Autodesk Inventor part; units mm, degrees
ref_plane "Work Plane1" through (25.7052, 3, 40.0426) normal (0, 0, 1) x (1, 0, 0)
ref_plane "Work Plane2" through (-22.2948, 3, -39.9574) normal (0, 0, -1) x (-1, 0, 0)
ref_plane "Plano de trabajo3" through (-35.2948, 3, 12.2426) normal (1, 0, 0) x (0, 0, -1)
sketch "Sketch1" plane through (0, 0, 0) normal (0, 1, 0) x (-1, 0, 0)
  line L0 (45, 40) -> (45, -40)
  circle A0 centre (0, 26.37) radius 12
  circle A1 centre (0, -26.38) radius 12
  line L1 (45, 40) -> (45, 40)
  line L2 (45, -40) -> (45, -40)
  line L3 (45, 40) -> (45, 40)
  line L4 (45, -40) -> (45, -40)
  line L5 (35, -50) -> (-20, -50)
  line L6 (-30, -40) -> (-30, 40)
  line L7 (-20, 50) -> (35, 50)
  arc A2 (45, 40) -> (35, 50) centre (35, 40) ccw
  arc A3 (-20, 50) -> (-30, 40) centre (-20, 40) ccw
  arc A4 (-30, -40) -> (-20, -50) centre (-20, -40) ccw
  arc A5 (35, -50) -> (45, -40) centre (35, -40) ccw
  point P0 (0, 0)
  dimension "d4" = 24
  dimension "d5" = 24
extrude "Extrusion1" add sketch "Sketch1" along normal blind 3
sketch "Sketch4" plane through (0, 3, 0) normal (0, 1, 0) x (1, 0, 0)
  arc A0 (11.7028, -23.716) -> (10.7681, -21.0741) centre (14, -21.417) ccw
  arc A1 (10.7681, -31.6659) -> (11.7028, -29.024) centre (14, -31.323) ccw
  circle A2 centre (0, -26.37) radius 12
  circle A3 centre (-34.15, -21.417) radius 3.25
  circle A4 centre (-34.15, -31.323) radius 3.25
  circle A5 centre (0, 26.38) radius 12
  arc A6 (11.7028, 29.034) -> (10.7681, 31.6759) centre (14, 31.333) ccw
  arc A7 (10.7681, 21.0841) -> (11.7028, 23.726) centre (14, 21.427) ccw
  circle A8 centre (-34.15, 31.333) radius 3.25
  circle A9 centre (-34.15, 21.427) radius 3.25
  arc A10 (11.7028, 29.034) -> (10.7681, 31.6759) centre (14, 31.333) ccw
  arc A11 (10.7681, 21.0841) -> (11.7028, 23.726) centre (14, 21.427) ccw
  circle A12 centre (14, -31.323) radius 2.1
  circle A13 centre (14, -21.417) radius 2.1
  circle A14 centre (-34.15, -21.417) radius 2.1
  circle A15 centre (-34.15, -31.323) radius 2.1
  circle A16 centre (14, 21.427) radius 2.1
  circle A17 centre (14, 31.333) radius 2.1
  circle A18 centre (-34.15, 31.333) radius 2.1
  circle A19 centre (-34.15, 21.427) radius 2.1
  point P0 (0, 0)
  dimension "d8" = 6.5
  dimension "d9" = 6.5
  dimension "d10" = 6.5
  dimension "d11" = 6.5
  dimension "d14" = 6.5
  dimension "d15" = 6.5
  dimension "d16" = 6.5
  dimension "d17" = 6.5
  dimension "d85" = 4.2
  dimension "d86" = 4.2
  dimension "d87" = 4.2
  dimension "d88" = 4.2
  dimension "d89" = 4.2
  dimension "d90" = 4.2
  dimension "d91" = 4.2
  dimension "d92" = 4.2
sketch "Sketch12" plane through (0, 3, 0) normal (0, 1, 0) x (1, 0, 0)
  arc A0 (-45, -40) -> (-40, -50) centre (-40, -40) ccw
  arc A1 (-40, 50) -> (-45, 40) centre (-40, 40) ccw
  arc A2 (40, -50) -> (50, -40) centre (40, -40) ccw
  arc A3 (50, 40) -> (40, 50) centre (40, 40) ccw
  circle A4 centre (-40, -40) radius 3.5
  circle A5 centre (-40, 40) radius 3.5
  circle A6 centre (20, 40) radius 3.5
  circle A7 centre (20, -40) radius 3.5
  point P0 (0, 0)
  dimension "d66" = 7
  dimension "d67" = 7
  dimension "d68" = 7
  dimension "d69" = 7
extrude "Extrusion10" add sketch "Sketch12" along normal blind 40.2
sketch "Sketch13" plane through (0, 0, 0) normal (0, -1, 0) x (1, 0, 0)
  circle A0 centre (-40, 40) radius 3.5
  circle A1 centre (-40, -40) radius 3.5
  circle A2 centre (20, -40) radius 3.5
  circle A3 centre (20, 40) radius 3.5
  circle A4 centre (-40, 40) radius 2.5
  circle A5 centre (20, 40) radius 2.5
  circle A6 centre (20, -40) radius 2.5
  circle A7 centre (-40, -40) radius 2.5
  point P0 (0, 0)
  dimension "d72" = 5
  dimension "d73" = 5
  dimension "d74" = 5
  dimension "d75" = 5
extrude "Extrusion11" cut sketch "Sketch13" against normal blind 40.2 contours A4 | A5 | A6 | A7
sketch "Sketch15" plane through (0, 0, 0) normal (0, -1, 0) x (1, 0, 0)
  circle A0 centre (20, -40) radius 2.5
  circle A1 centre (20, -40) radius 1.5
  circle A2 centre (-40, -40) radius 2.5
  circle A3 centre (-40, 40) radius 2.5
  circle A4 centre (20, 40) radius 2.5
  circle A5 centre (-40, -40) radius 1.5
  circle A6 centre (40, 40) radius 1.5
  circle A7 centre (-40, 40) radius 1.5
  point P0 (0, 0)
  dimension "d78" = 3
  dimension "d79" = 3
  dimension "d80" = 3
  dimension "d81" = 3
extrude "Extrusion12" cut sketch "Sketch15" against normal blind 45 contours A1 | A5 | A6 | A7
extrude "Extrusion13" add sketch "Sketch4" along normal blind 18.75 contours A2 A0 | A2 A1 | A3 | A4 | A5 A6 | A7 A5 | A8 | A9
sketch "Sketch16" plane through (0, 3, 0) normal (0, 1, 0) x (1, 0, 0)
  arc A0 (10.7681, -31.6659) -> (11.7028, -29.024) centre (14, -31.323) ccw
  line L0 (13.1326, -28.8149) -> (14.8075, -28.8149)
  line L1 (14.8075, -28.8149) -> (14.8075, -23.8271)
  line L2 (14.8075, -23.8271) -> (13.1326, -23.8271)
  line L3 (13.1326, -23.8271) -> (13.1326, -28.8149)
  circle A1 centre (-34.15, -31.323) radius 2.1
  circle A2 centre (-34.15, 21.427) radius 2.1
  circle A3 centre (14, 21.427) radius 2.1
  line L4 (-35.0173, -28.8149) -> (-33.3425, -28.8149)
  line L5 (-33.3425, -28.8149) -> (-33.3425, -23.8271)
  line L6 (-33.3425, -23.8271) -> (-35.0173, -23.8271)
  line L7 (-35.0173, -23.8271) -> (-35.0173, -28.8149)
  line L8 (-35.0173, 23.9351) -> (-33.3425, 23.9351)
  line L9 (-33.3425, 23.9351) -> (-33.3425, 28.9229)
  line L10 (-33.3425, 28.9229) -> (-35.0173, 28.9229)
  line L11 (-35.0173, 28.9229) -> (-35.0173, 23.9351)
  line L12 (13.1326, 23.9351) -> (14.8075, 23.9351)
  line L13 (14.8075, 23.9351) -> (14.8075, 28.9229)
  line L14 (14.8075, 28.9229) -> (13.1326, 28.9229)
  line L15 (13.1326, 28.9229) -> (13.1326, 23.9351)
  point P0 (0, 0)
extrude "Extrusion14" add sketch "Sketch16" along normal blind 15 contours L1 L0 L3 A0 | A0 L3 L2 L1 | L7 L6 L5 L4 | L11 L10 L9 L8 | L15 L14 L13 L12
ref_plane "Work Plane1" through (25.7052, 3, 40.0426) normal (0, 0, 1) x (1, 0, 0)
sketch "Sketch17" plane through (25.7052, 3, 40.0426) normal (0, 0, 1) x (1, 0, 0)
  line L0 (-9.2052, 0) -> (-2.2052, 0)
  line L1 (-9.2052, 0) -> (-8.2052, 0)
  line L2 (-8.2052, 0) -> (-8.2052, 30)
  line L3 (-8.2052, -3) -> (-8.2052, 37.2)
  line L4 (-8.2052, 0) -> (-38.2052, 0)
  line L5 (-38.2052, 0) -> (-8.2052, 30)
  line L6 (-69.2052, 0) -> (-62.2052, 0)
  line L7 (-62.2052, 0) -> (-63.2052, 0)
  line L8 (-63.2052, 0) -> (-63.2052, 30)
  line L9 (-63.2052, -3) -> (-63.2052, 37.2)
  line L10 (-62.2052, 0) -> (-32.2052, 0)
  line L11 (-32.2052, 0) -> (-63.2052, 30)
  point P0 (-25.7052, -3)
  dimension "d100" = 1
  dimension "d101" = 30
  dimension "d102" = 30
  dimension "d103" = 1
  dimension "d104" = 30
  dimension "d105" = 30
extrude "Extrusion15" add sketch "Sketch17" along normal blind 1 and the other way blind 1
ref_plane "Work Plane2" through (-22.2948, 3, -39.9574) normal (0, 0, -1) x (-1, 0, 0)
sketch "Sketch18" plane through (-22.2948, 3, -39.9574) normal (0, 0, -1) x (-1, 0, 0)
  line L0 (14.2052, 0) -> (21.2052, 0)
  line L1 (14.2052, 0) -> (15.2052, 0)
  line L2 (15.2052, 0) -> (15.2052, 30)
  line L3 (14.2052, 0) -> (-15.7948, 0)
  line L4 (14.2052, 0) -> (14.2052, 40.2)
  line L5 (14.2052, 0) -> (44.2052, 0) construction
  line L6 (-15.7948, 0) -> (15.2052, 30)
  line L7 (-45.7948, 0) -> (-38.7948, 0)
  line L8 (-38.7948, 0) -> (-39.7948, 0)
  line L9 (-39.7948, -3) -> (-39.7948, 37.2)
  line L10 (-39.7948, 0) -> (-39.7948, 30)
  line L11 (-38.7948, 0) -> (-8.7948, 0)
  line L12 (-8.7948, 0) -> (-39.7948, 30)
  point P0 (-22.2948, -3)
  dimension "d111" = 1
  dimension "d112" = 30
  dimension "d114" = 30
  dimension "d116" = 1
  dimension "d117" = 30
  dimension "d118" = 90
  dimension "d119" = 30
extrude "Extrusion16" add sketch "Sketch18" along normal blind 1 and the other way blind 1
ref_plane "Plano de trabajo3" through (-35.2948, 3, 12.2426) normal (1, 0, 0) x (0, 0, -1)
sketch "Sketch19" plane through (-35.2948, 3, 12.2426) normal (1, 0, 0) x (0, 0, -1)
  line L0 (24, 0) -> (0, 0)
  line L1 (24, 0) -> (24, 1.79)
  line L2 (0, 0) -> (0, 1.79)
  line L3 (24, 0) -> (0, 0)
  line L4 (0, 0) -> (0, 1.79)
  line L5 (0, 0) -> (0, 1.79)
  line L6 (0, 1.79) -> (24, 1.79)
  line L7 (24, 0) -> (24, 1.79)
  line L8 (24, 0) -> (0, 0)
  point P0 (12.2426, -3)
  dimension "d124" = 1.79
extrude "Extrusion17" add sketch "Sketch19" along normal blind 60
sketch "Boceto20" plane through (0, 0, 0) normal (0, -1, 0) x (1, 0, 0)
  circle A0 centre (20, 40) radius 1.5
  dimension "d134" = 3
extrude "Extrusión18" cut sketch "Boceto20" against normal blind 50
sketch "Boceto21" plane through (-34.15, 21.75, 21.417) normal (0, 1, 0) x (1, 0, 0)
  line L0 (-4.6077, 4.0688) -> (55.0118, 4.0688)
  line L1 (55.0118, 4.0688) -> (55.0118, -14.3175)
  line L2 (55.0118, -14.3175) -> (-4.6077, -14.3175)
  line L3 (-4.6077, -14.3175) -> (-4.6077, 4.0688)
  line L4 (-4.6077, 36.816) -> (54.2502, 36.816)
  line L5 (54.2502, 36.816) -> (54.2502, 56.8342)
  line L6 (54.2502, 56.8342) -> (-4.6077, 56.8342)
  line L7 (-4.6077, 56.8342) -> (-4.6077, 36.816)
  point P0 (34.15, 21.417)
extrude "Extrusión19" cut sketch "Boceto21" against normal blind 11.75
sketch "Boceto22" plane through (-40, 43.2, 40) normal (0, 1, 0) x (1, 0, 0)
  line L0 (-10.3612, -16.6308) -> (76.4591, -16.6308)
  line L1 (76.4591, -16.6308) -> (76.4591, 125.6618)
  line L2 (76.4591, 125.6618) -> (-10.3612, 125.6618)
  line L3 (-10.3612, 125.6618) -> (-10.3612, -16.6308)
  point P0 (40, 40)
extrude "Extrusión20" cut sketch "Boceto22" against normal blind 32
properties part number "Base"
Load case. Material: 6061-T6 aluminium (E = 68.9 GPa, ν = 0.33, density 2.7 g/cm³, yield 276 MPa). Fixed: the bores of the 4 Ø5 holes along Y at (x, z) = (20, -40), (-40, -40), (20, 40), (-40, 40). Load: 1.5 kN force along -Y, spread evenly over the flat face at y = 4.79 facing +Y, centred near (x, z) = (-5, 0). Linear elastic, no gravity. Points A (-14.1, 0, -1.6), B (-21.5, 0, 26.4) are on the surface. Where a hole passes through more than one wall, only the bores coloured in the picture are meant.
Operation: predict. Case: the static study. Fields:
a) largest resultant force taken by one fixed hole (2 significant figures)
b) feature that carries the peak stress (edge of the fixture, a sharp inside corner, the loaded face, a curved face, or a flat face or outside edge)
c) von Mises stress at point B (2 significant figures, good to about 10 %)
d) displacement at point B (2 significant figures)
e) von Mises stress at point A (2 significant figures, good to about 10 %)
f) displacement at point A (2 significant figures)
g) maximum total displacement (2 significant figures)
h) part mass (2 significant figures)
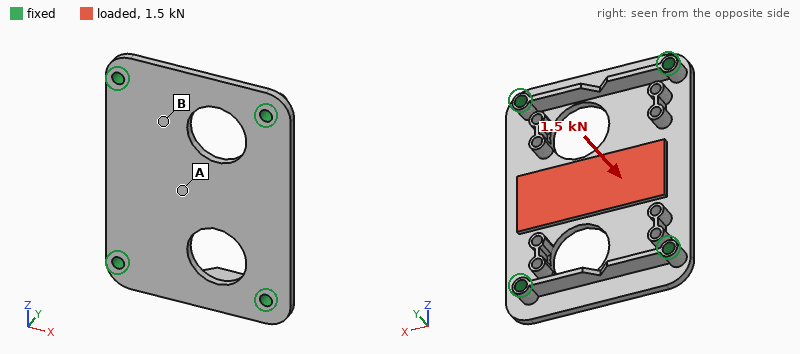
470 N
a flat face or outside edge
18 MPa
0.13 mm
43 MPa
0.27 mm
0.28 mm
68 g
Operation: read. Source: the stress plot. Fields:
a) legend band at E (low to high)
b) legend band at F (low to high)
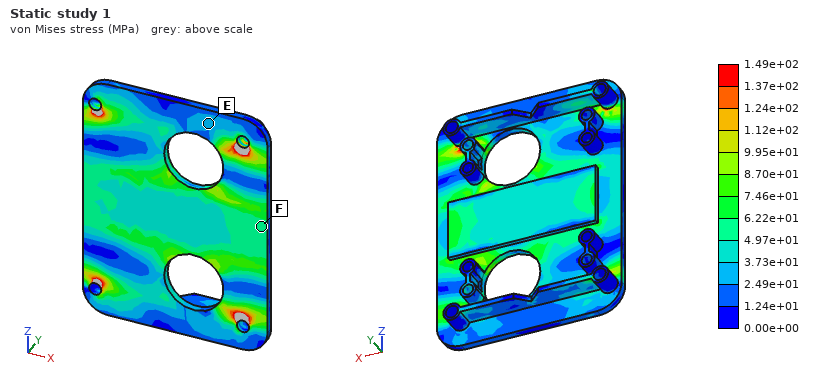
2.49e+01 to 3.73e+01 MPa
4.97e+01 to 6.22e+01 MPa
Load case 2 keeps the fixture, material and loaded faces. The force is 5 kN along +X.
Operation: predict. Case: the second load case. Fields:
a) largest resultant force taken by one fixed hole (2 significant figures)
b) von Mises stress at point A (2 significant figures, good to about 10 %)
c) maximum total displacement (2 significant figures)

1.9 kN
13 MPa
0.14 mm
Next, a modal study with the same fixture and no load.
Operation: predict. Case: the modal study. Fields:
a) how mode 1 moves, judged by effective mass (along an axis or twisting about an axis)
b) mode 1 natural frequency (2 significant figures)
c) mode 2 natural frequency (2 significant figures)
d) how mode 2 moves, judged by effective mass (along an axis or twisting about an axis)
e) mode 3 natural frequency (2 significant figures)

along Y
2200 Hz
3100 Hz
twisting about Z
5900 Hz
